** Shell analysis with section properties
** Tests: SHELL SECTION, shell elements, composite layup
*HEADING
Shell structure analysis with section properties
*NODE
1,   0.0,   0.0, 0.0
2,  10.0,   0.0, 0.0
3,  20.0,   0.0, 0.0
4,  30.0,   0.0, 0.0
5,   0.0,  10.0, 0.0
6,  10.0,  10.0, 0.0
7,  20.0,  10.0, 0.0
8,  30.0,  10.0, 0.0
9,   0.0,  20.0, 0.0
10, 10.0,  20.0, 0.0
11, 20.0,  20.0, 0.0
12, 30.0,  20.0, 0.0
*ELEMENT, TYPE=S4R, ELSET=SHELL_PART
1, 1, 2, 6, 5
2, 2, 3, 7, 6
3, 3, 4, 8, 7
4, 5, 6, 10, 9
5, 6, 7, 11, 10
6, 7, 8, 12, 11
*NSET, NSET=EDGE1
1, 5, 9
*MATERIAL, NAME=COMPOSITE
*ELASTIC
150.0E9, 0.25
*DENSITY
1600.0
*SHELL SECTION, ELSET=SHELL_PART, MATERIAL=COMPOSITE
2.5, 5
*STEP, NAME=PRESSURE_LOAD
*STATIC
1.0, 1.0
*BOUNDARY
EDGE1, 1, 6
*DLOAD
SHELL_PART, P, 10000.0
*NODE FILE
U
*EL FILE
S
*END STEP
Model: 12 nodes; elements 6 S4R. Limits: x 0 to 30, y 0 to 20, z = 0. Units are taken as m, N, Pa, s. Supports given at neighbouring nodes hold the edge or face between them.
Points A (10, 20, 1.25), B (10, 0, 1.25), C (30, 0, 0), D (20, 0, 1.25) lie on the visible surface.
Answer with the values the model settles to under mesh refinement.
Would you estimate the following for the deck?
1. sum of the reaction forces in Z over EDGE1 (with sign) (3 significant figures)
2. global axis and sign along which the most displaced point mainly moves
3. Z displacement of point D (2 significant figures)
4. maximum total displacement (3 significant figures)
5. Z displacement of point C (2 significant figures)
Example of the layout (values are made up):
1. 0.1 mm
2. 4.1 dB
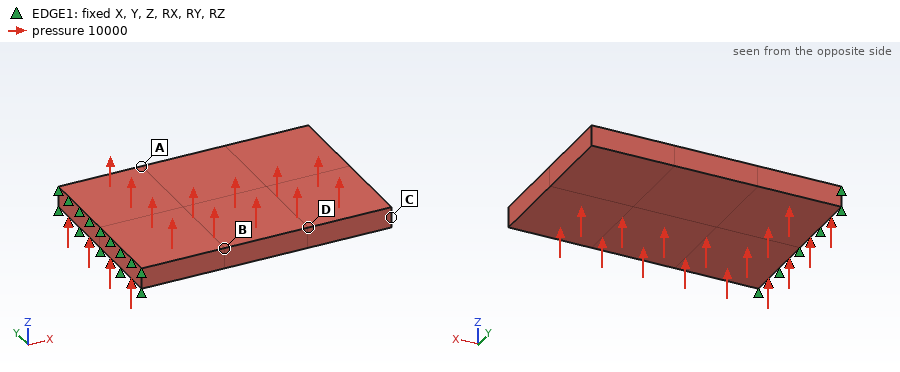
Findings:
1. -6.00e+06 N
2. +Z
3. 0.0027 m
4. 0.00495 m
5. 0.0049 m
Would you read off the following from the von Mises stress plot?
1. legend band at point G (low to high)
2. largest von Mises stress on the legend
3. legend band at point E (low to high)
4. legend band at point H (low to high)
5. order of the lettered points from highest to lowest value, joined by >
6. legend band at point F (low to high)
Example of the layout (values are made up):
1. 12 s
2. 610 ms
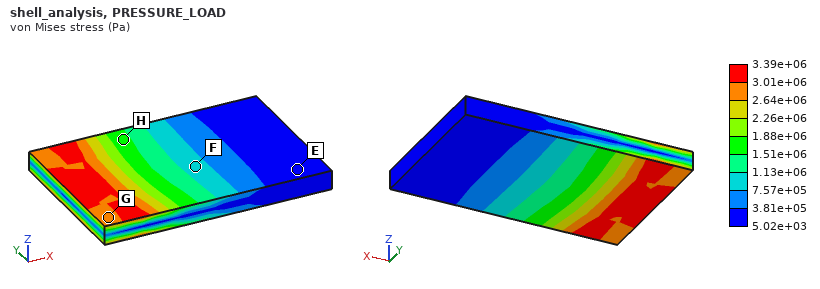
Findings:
1. 2.64e+06 to 3.01e+06 Pa
2. 3.39e+06 Pa
3. 5.02e+03 to 3.81e+05 Pa
4. 1.51e+06 to 1.88e+06 Pa
5. G > H > F > E
6. 7.57e+05 to 1.13e+06 Pa
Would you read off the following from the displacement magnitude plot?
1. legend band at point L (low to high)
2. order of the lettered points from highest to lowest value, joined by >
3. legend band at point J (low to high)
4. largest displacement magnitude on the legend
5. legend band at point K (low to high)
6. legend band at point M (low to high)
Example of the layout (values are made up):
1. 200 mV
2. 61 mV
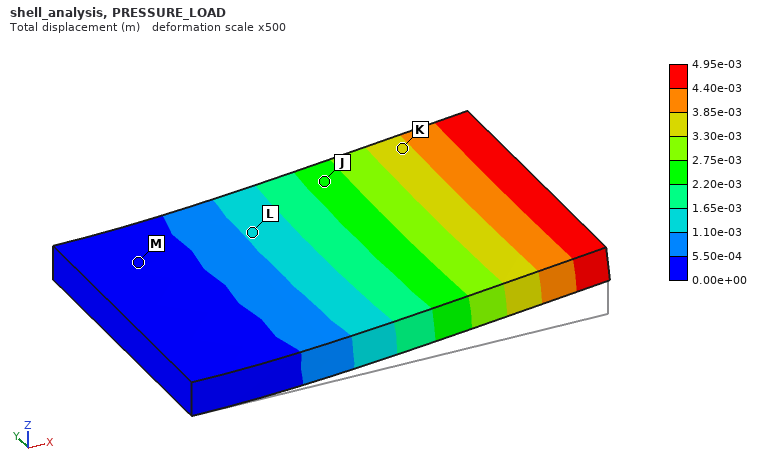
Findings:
1. 1.10e-03 to 1.65e-03 m
2. K > J > L > M
3. 2.20e-03 to 2.75e-03 m
4. 4.95e-03 m
5. 3.30e-03 to 3.85e-03 m
6. 0.00e+00 to 5.50e-04 m
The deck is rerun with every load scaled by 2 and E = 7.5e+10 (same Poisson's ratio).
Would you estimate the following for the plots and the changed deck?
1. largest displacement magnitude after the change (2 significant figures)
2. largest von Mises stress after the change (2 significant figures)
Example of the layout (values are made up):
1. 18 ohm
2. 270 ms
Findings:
1. 0.020 m
2. 6.8e+06 Pa
